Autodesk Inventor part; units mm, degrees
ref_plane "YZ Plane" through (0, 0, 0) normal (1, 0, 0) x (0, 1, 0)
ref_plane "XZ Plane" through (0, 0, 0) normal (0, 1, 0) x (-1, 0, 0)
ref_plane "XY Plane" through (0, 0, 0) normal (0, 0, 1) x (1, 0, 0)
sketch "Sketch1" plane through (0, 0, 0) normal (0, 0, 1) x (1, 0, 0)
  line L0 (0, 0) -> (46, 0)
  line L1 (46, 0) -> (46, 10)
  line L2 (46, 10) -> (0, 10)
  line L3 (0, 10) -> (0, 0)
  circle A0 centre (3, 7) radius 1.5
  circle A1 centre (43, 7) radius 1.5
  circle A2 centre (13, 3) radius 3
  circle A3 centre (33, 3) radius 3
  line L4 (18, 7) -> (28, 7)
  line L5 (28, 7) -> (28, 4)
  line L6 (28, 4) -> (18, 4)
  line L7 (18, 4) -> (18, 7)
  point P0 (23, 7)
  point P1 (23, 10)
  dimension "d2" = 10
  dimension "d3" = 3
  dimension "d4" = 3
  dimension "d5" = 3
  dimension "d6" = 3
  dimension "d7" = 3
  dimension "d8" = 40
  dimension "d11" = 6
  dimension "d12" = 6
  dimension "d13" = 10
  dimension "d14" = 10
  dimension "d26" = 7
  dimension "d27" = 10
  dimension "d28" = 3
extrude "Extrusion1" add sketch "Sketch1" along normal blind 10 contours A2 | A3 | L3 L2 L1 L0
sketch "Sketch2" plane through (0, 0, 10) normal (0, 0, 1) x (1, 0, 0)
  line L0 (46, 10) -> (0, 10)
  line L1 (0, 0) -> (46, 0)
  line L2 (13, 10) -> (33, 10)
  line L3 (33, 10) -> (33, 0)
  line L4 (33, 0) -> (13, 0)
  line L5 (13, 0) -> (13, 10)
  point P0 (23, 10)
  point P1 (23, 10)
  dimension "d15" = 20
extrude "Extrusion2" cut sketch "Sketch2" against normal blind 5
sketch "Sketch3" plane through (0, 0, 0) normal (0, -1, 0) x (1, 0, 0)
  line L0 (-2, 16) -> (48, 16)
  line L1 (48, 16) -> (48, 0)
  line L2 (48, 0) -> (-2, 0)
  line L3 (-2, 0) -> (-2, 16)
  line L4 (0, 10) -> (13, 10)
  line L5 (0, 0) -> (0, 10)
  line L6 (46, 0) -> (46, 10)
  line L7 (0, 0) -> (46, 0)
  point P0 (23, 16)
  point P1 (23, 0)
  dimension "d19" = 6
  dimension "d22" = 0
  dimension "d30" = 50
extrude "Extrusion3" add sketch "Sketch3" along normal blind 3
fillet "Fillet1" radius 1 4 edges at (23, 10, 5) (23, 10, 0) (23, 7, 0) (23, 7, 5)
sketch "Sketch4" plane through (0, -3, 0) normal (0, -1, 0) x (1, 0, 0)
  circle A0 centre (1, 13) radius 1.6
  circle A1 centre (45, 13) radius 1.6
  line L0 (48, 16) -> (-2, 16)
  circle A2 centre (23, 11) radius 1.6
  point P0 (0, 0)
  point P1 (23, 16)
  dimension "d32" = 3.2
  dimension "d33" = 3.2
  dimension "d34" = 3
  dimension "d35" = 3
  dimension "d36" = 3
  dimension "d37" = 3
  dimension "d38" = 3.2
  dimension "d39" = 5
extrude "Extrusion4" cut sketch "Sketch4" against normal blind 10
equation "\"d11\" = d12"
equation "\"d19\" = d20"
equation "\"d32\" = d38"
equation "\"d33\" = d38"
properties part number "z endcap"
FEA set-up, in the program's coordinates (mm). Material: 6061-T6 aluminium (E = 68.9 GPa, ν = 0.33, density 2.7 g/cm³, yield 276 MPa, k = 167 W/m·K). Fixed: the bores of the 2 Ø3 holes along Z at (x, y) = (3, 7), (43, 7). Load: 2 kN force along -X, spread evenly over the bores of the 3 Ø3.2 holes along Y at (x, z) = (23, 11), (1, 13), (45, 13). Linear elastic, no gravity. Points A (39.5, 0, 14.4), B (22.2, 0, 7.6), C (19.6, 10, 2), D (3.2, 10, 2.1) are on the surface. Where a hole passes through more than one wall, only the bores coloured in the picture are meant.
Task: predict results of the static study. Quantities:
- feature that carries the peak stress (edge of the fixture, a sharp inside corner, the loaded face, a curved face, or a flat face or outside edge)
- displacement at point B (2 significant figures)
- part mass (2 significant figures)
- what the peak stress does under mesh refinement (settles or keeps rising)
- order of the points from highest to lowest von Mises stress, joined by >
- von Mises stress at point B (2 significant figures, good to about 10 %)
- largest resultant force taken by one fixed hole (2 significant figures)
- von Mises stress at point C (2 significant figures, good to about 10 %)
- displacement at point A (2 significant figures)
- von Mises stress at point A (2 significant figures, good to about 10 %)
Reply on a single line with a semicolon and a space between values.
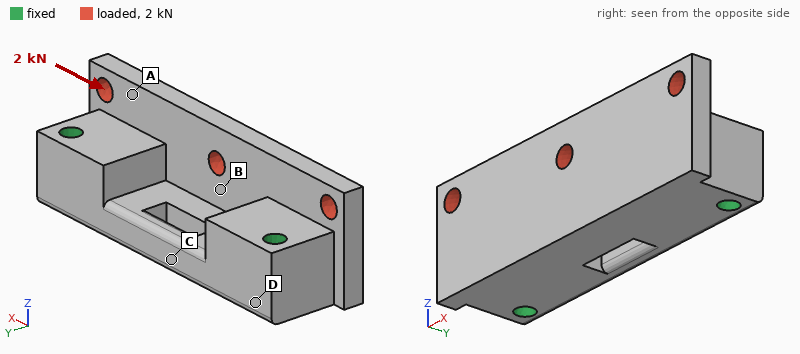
edge of the fixture; 6.9 µm; 15 g; keeps rising; B > A > C > D; 33 MPa; 1.1 kN; 15 MPa; 11 µm; 22 MPa
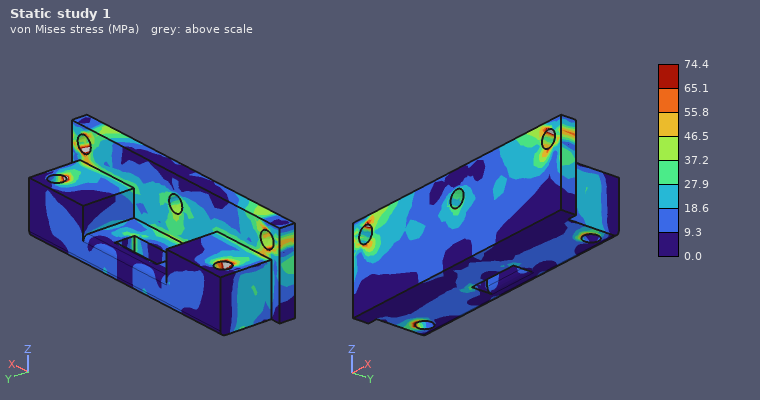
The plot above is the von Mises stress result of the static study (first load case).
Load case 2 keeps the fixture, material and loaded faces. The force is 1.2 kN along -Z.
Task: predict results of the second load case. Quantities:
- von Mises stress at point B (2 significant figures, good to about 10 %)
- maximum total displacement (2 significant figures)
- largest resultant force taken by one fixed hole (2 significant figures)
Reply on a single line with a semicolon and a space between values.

11 MPa; 11 µm; 600 N
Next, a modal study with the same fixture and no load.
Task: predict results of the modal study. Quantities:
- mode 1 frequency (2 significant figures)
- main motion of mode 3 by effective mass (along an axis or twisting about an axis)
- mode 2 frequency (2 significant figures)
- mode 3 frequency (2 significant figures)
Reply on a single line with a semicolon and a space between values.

18 kHz; along X; 23 kHz; 25 kHz
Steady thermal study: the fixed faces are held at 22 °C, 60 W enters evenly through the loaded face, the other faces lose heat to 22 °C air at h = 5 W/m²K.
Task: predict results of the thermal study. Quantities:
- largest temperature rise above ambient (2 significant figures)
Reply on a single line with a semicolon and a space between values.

46 K
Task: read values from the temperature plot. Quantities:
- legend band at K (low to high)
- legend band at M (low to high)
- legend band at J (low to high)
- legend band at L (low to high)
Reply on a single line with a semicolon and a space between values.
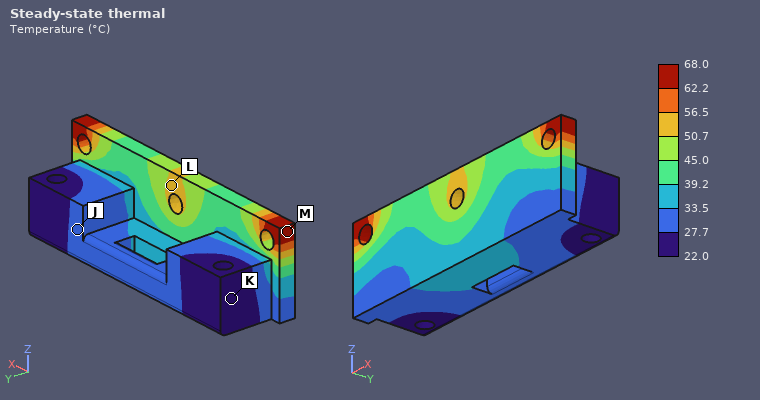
22.0 to 27.7 °C; 62.2 to 68.0 °C; 27.7 to 33.5 °C; 50.7 to 56.5 °C
